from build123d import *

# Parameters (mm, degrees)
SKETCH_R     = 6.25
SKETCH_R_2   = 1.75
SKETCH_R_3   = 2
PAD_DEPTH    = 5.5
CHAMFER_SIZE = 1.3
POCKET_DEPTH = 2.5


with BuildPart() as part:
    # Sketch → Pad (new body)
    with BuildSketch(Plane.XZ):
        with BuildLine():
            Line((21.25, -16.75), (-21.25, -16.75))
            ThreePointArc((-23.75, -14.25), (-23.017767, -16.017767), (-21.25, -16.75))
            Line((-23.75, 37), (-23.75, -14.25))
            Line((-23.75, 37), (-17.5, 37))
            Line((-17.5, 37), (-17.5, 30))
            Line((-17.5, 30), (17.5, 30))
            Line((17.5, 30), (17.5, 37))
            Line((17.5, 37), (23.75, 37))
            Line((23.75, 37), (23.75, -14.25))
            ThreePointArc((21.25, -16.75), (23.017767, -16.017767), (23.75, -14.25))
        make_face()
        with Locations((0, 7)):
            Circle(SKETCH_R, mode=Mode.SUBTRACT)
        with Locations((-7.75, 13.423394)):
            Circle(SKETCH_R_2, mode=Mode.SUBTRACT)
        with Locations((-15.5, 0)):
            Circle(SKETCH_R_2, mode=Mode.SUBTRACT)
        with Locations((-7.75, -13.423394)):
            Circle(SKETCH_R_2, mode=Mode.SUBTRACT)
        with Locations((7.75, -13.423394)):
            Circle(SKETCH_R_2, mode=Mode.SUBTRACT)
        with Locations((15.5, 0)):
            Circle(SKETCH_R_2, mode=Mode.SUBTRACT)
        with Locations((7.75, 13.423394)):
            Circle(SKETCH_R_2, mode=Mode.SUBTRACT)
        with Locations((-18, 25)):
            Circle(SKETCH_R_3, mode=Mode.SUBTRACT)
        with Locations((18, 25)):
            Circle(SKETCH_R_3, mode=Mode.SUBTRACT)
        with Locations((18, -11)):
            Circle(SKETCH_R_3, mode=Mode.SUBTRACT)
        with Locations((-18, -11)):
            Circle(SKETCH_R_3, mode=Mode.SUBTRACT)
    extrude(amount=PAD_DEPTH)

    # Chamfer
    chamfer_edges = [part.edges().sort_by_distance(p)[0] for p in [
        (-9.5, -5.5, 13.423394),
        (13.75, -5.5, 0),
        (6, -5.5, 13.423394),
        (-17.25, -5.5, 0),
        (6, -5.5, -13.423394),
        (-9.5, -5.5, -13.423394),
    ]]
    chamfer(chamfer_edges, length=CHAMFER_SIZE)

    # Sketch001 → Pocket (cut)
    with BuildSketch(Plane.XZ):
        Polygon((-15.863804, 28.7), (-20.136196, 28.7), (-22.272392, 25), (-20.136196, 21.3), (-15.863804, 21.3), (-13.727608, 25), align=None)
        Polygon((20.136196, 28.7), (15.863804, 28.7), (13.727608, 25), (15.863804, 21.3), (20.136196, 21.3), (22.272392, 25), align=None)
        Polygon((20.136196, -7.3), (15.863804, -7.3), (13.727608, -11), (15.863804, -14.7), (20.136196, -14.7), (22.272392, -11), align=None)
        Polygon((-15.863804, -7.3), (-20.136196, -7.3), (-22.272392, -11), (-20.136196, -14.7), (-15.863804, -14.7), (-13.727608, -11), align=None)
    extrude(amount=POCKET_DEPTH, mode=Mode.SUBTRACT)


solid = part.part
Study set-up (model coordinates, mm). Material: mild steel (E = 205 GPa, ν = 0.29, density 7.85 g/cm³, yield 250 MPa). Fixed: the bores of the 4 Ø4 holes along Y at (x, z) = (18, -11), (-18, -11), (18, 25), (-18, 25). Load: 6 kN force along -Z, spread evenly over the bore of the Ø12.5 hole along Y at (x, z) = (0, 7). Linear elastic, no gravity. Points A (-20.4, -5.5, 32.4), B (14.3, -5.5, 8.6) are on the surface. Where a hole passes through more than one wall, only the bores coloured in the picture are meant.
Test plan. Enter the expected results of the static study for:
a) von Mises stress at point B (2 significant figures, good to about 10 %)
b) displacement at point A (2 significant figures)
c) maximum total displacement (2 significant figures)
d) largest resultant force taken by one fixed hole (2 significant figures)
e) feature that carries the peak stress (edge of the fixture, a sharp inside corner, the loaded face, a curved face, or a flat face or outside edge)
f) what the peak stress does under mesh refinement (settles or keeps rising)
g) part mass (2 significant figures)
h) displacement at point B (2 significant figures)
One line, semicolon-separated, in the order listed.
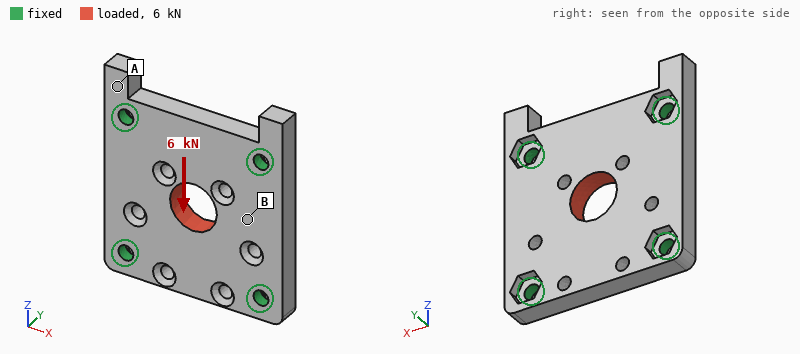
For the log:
18 MPa; 0.90 µm; 4.6 µm; 1.6 kN; edge of the fixture; keeps rising; 86 g; 2.1 µm
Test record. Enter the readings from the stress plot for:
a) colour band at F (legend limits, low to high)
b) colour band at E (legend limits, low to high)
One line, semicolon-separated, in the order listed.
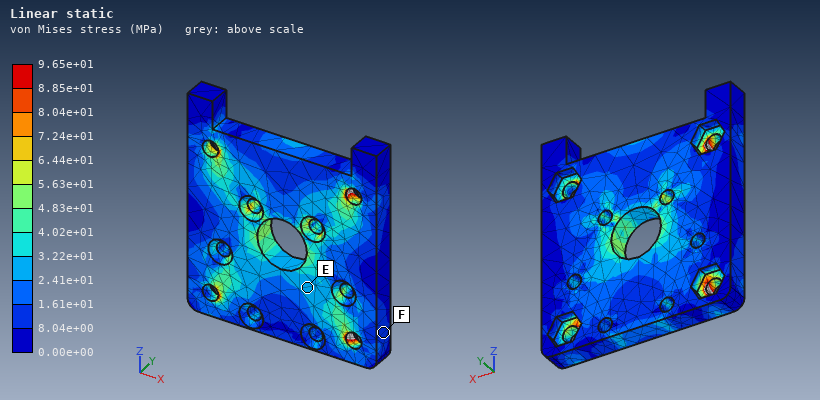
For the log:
8.04e+00 to 1.61e+01 MPa; 2.41e+01 to 3.22e+01 MPa
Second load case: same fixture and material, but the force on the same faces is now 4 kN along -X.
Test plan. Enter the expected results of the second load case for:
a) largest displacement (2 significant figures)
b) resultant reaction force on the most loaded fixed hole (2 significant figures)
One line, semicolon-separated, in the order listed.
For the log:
3.1 µm; 1.1 kN
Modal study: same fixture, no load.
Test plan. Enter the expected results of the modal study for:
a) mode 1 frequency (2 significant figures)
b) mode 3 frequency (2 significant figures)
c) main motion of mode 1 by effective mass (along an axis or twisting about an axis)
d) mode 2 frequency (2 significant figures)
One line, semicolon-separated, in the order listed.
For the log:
12 kHz; 18 kHz; along Y; 18 kHz
